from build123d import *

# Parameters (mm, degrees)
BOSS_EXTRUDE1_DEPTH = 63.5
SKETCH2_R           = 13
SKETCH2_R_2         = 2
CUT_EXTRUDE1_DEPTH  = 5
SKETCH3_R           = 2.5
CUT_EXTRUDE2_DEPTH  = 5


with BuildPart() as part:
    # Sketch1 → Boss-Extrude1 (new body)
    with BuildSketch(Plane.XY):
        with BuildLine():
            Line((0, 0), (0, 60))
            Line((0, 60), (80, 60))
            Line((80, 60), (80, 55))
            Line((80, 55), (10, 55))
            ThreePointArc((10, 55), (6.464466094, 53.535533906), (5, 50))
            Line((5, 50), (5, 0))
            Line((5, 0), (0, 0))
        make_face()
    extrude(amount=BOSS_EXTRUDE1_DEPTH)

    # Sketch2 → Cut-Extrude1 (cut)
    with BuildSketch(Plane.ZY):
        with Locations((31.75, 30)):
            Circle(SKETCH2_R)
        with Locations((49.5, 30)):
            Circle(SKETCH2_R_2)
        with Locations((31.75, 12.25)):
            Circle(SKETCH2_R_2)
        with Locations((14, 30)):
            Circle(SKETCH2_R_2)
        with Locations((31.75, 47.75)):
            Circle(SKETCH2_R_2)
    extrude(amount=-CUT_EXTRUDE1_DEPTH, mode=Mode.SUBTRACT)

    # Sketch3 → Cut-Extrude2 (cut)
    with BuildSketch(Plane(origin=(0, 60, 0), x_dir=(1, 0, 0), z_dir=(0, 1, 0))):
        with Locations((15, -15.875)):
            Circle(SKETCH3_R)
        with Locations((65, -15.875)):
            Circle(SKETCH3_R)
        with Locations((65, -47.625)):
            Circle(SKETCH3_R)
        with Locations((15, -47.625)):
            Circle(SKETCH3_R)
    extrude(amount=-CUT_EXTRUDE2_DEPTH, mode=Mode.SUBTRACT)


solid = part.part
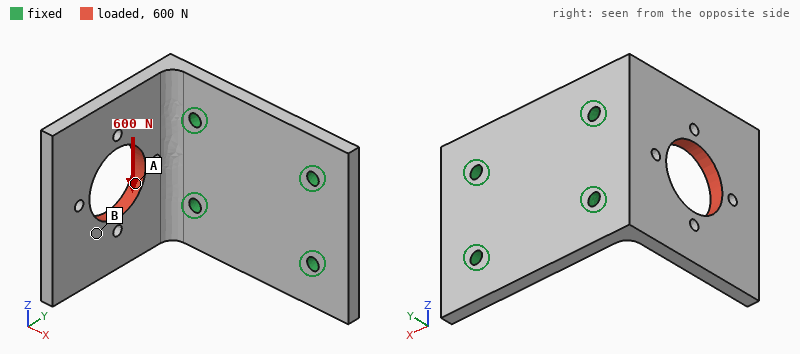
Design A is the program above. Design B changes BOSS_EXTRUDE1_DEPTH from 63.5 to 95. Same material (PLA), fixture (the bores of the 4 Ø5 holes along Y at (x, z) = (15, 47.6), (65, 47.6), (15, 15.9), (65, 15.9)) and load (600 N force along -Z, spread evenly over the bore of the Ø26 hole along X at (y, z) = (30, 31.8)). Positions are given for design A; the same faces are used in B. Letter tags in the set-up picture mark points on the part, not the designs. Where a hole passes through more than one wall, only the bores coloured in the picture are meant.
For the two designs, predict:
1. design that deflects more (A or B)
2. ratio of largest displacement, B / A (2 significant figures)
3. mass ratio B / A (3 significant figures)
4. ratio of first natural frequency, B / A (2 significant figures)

B
1.2
1.54
0.95
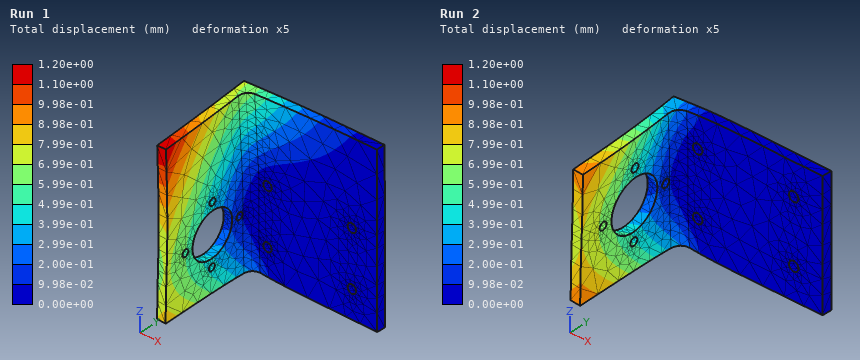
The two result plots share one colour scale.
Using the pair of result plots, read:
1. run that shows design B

Run 1
